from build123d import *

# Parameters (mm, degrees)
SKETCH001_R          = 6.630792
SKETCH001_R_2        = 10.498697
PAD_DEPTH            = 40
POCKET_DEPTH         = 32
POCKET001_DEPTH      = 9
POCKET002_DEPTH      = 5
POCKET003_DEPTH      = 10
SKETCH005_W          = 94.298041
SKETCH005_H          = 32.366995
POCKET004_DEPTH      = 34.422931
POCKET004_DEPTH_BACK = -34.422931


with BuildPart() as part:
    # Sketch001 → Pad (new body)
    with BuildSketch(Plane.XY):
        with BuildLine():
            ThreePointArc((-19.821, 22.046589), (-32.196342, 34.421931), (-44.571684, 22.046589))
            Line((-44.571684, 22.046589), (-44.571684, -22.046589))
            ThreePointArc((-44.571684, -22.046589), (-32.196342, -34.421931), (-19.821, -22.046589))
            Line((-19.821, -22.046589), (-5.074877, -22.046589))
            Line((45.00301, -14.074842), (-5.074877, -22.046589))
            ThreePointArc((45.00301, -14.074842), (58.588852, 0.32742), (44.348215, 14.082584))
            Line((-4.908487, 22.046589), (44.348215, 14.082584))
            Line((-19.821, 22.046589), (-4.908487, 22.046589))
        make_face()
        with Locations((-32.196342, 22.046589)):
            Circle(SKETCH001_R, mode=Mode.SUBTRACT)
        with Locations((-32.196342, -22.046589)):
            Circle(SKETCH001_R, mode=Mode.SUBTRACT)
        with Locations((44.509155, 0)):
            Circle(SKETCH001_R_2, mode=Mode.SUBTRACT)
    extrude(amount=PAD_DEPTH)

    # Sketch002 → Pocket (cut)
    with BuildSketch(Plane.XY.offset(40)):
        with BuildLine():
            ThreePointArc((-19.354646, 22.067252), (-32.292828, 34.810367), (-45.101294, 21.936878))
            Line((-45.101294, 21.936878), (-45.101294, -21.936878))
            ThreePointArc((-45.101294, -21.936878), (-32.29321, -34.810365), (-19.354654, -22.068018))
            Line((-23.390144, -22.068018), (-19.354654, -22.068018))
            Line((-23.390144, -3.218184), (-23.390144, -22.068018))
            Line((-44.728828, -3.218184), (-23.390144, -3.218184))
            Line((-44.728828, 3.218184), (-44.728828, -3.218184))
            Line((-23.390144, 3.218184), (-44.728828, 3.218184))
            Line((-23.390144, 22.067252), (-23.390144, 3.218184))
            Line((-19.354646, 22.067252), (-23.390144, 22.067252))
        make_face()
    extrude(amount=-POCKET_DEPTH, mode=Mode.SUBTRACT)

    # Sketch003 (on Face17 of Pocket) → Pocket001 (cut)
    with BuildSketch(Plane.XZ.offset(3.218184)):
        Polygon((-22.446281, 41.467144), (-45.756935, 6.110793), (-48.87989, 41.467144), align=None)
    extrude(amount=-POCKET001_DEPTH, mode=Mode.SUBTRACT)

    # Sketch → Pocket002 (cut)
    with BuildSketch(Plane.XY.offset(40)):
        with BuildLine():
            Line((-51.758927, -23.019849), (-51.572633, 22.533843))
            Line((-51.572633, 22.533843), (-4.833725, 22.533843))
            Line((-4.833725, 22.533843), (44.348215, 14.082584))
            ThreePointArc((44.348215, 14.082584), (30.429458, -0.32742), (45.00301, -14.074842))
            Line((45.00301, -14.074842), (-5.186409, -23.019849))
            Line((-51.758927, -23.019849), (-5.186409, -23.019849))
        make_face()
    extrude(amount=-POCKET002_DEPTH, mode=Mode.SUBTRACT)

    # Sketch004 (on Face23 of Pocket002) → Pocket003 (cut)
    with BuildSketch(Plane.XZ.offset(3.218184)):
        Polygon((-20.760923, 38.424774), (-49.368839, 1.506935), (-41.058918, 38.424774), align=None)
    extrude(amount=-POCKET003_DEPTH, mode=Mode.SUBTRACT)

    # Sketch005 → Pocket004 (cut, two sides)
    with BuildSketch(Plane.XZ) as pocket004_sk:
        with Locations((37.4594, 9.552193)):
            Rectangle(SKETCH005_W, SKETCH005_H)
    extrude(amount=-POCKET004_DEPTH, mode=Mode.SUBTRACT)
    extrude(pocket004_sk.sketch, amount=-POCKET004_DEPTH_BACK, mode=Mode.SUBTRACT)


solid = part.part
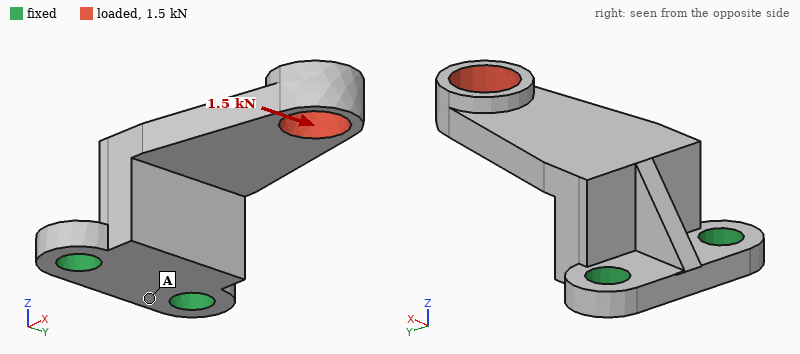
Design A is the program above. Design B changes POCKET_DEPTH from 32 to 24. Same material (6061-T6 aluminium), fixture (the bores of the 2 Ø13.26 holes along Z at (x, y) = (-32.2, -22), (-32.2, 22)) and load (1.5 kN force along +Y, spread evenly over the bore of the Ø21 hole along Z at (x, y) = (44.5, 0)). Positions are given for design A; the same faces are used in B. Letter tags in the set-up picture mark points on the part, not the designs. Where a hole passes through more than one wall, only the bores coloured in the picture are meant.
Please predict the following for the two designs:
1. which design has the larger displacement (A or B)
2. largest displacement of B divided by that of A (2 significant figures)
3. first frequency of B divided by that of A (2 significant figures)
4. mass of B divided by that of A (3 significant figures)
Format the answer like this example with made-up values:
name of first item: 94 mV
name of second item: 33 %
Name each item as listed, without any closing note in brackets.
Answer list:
which design has the larger displacement: A
largest displacement of B divided by that of A: 0.71
first frequency of B divided by that of A: 1.2
mass of B divided by that of A: 1.15
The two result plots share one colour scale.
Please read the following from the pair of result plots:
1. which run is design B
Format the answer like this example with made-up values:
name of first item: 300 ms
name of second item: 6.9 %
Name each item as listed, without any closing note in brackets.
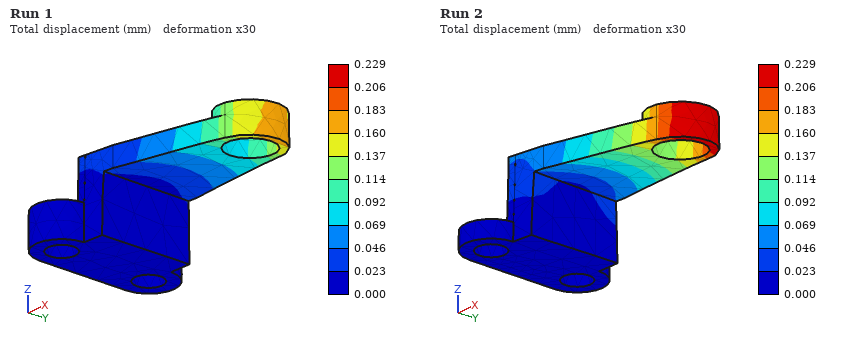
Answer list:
which run is design B: Run 1
